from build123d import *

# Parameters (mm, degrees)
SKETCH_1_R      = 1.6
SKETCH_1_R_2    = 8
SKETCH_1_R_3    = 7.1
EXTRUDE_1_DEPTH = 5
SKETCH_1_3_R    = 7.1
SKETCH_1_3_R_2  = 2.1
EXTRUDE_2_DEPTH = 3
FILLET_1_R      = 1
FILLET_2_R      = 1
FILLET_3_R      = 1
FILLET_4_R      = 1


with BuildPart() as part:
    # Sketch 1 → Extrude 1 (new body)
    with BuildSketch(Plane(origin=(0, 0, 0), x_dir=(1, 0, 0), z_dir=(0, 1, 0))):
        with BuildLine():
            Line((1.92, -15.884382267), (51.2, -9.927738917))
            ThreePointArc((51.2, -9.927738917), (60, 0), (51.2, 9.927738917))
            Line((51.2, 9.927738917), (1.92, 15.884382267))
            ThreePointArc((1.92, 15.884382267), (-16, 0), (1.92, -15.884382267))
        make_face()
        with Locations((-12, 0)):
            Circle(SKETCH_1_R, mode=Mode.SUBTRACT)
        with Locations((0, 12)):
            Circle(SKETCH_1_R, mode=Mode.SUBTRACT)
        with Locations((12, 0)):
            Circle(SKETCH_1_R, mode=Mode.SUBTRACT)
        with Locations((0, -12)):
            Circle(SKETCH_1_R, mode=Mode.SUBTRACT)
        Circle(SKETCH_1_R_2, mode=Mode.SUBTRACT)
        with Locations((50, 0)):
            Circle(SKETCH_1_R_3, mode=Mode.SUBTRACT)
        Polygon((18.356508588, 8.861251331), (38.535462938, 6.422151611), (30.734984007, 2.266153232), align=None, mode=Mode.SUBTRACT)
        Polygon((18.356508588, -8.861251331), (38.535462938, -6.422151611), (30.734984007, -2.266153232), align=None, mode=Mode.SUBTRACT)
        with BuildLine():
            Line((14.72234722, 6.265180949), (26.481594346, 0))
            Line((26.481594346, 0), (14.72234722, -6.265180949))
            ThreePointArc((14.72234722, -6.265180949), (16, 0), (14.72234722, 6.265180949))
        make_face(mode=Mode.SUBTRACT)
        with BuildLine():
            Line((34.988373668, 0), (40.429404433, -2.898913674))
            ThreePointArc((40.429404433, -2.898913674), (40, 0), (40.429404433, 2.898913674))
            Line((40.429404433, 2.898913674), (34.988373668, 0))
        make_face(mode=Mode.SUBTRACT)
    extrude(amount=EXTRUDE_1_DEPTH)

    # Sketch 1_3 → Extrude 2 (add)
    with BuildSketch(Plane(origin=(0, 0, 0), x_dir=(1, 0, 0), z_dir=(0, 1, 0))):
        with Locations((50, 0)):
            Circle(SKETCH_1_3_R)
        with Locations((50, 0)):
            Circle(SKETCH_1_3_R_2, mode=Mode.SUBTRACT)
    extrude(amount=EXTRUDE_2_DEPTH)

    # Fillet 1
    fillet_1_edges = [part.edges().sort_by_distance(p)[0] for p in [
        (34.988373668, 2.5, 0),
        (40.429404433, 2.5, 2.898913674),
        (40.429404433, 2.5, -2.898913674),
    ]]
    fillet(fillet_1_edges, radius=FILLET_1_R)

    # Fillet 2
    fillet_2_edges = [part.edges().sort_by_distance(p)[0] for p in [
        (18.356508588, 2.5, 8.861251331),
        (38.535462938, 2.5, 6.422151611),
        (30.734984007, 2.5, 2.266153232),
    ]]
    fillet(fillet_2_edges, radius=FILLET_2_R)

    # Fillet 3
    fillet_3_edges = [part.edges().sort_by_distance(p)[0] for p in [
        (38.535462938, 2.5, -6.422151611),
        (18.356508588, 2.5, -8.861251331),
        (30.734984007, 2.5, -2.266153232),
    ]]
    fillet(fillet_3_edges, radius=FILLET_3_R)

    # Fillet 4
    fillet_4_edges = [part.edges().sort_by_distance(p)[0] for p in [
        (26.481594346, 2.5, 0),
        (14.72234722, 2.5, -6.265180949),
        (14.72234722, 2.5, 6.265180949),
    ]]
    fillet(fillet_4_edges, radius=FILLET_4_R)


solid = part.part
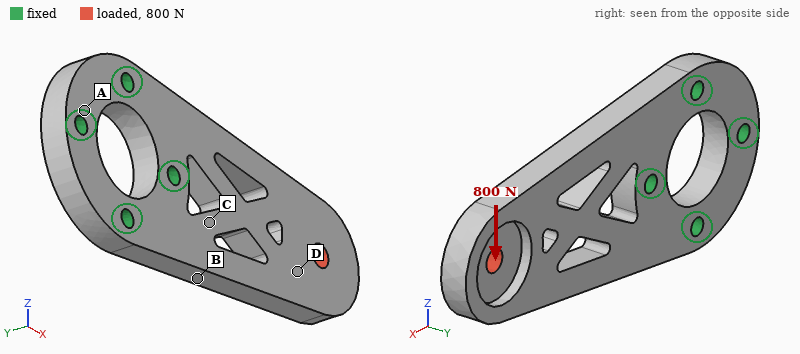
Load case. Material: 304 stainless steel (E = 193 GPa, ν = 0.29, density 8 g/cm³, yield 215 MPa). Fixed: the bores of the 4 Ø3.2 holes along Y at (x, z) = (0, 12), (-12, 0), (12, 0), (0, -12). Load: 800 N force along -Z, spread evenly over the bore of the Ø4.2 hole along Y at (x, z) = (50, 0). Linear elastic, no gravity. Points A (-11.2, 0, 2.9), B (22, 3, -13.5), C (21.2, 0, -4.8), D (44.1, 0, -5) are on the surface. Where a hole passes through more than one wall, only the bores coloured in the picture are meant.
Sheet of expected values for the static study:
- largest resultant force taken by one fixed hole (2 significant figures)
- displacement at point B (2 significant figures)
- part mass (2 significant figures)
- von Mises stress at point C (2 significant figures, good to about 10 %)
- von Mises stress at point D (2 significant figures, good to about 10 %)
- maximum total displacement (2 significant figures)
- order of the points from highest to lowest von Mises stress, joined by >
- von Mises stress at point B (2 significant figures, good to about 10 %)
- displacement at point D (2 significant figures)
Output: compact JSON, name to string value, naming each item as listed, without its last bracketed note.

{"largest resultant force taken by one fixed hole": "1.2 kN", "displacement at point B": "6.9 µm", "part mass": "56 g", "von Mises stress at point C": "32 MPa", "von Mises stress at point D": "23 MPa", "maximum total displacement": "31 µm", "order of the points from highest to lowest von Mises stress, joined by >": "B > C > D > A", "von Mises stress at point B": "51 MPa", "displacement at point D": "21 µm"}
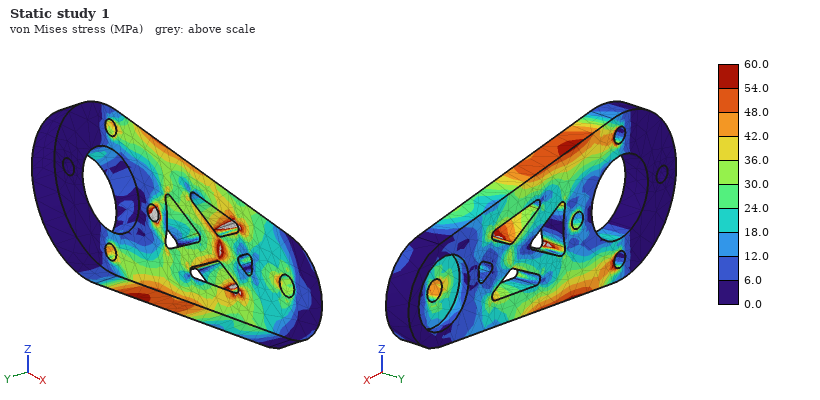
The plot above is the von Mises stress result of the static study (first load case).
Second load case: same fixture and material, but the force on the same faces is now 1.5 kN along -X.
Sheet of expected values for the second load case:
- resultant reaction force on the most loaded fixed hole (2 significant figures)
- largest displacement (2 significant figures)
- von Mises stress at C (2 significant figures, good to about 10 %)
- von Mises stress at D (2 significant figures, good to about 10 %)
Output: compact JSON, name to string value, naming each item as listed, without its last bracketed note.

{"resultant reaction force on the most loaded fixed hole": "540 N", "largest displacement": "52 µm", "von Mises stress at C": "37 MPa", "von Mises stress at D": "32 MPa"}
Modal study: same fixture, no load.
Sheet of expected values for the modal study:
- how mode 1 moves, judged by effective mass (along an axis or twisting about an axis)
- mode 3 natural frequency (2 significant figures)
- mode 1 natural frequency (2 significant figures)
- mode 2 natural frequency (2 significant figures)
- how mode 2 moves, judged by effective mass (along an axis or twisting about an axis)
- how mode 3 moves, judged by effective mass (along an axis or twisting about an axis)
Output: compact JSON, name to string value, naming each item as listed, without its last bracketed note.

{"how mode 1 moves, judged by effective mass": "along Y", "mode 3 natural frequency": "7500 Hz", "mode 1 natural frequency": "1700 Hz", "mode 2 natural frequency": "6200 Hz", "how mode 2 moves, judged by effective mass": "twisting about X", "how mode 3 moves, judged by effective mass": "along Z"}
